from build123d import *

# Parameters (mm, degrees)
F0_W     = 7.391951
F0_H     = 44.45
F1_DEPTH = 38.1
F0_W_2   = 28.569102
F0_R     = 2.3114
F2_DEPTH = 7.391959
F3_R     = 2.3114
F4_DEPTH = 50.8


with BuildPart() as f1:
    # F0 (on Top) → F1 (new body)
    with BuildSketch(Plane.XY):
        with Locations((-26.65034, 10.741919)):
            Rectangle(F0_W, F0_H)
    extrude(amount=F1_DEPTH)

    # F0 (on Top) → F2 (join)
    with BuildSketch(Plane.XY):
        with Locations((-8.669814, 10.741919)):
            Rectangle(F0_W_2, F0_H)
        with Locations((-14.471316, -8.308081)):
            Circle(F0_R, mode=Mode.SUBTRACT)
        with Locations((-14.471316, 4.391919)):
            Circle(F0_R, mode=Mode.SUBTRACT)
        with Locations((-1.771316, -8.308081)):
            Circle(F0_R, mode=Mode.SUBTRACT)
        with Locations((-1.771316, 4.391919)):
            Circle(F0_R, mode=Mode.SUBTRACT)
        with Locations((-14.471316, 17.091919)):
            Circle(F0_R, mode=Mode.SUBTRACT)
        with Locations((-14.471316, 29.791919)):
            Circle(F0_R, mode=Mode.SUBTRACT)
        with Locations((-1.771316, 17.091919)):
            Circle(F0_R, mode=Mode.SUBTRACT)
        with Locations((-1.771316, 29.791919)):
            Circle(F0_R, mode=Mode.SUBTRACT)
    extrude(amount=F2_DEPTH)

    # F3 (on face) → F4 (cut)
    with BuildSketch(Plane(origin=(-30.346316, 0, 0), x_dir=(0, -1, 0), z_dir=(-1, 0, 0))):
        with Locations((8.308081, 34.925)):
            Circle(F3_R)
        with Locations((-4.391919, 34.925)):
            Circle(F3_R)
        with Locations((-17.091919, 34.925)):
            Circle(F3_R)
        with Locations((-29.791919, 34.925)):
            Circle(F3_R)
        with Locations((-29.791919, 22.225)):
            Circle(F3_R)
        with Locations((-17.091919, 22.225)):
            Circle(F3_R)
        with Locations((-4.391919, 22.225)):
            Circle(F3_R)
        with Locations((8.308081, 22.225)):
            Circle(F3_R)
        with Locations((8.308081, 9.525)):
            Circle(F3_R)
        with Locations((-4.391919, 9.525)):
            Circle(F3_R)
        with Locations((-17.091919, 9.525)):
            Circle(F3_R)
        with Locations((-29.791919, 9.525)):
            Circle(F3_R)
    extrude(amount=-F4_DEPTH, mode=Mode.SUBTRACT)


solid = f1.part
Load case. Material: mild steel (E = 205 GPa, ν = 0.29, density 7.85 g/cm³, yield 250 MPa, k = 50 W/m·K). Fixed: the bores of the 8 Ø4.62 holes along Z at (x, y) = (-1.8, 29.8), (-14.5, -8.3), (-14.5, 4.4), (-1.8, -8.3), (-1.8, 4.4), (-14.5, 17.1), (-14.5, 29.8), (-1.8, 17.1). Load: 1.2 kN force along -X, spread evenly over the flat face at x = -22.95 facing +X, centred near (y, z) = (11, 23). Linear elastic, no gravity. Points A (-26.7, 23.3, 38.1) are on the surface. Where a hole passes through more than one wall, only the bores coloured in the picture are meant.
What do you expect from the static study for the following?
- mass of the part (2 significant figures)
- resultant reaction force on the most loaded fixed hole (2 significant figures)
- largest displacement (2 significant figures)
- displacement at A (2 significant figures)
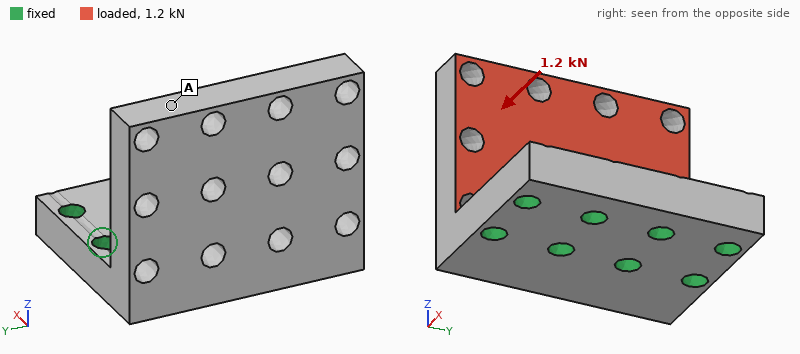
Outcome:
150 g
390 N
53 µm
52 µm
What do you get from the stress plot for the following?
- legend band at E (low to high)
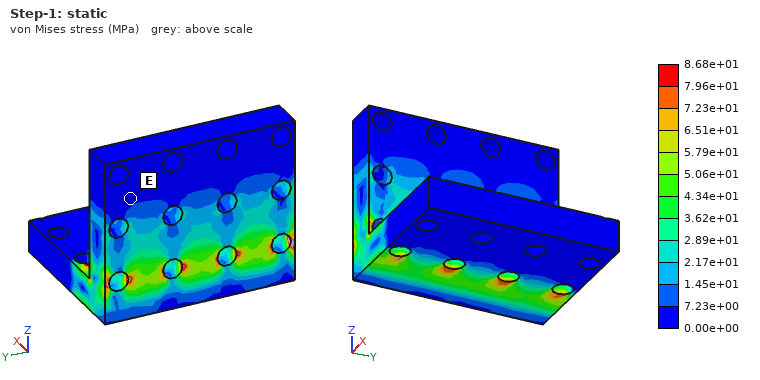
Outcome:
0.00e+00 to 7.23e+00 MPa
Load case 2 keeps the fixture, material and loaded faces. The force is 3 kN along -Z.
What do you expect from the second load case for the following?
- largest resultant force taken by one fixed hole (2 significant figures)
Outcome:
940 N
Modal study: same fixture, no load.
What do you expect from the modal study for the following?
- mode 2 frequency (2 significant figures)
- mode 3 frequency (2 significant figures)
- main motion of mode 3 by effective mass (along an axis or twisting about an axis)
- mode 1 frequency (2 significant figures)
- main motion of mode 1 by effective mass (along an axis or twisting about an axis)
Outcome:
7400 Hz
9800 Hz
along Y
3600 Hz
along X
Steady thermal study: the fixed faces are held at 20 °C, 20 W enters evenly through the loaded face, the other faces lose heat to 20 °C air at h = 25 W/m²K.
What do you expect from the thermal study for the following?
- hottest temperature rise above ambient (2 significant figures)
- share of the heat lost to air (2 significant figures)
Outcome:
35 K
13 %
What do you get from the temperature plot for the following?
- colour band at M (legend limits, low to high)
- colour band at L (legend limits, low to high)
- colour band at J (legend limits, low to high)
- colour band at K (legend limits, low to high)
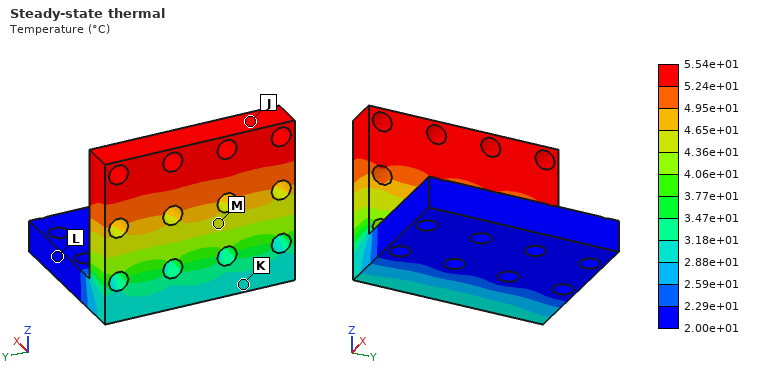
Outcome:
4.36e+01 to 4.65e+01 °C
2.00e+01 to 2.29e+01 °C
5.24e+01 to 5.54e+01 °C
2.88e+01 to 3.18e+01 °C
